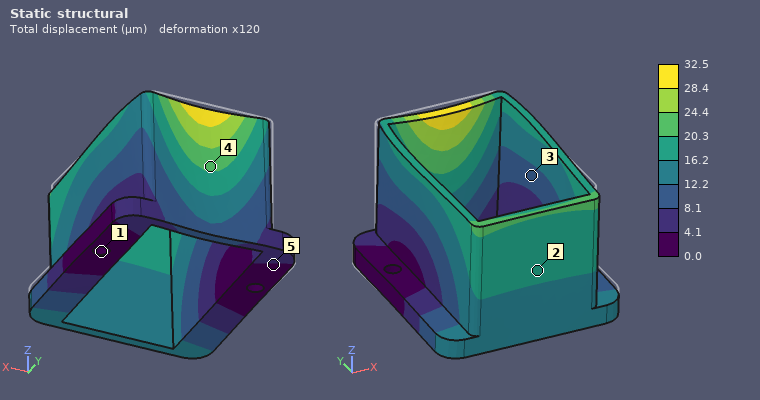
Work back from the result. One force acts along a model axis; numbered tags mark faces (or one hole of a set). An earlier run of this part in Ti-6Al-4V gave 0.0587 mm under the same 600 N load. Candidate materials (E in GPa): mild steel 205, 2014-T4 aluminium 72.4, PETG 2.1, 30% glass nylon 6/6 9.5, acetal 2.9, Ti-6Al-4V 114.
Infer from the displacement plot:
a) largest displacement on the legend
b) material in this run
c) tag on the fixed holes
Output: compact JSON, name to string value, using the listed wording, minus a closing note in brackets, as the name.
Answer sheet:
{"largest displacement on the legend": "32.5 µm", "material in this run": "mild steel", "tag on the fixed holes": "1"}
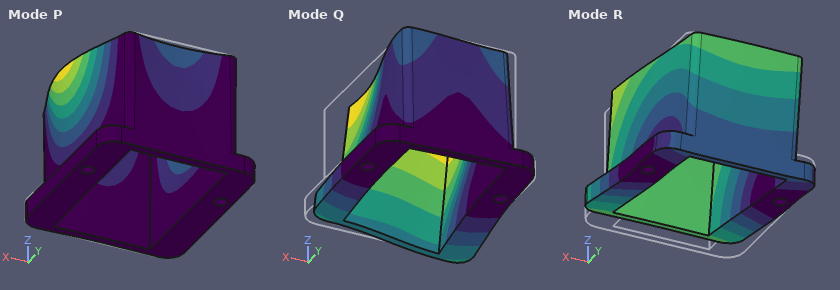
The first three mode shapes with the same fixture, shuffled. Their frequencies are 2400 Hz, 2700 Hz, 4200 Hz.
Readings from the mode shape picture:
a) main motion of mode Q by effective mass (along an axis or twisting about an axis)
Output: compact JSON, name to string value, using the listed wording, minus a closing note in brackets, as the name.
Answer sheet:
{"main motion of mode Q by effective mass": "along X"}
